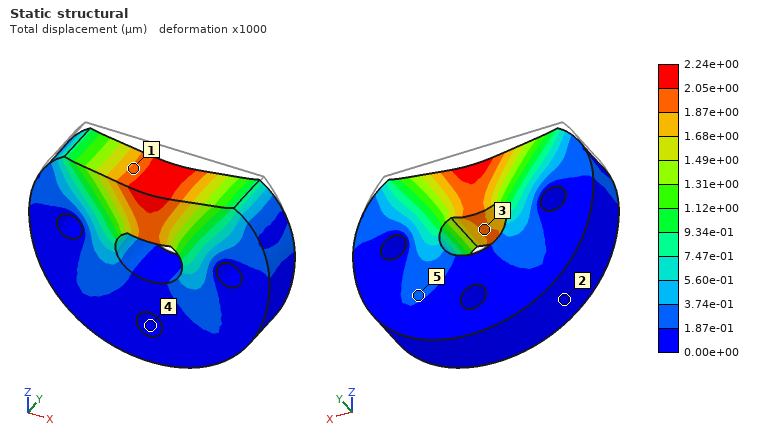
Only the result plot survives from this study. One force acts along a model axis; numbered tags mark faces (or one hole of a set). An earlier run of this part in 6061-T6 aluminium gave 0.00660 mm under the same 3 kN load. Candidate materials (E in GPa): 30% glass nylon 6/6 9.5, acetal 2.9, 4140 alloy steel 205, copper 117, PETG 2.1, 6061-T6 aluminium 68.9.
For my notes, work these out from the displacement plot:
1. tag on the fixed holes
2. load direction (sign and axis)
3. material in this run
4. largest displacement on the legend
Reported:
4
-Z
4140 alloy steel
2.24e+00 µm
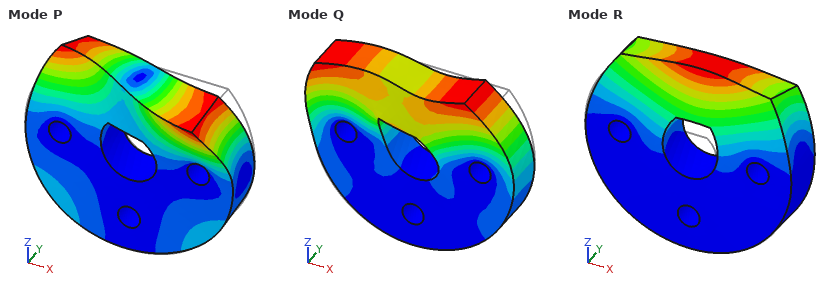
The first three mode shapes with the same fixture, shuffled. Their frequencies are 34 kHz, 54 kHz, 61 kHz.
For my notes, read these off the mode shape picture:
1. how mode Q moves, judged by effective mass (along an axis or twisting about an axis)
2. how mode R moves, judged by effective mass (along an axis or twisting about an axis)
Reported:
along X
along Y
